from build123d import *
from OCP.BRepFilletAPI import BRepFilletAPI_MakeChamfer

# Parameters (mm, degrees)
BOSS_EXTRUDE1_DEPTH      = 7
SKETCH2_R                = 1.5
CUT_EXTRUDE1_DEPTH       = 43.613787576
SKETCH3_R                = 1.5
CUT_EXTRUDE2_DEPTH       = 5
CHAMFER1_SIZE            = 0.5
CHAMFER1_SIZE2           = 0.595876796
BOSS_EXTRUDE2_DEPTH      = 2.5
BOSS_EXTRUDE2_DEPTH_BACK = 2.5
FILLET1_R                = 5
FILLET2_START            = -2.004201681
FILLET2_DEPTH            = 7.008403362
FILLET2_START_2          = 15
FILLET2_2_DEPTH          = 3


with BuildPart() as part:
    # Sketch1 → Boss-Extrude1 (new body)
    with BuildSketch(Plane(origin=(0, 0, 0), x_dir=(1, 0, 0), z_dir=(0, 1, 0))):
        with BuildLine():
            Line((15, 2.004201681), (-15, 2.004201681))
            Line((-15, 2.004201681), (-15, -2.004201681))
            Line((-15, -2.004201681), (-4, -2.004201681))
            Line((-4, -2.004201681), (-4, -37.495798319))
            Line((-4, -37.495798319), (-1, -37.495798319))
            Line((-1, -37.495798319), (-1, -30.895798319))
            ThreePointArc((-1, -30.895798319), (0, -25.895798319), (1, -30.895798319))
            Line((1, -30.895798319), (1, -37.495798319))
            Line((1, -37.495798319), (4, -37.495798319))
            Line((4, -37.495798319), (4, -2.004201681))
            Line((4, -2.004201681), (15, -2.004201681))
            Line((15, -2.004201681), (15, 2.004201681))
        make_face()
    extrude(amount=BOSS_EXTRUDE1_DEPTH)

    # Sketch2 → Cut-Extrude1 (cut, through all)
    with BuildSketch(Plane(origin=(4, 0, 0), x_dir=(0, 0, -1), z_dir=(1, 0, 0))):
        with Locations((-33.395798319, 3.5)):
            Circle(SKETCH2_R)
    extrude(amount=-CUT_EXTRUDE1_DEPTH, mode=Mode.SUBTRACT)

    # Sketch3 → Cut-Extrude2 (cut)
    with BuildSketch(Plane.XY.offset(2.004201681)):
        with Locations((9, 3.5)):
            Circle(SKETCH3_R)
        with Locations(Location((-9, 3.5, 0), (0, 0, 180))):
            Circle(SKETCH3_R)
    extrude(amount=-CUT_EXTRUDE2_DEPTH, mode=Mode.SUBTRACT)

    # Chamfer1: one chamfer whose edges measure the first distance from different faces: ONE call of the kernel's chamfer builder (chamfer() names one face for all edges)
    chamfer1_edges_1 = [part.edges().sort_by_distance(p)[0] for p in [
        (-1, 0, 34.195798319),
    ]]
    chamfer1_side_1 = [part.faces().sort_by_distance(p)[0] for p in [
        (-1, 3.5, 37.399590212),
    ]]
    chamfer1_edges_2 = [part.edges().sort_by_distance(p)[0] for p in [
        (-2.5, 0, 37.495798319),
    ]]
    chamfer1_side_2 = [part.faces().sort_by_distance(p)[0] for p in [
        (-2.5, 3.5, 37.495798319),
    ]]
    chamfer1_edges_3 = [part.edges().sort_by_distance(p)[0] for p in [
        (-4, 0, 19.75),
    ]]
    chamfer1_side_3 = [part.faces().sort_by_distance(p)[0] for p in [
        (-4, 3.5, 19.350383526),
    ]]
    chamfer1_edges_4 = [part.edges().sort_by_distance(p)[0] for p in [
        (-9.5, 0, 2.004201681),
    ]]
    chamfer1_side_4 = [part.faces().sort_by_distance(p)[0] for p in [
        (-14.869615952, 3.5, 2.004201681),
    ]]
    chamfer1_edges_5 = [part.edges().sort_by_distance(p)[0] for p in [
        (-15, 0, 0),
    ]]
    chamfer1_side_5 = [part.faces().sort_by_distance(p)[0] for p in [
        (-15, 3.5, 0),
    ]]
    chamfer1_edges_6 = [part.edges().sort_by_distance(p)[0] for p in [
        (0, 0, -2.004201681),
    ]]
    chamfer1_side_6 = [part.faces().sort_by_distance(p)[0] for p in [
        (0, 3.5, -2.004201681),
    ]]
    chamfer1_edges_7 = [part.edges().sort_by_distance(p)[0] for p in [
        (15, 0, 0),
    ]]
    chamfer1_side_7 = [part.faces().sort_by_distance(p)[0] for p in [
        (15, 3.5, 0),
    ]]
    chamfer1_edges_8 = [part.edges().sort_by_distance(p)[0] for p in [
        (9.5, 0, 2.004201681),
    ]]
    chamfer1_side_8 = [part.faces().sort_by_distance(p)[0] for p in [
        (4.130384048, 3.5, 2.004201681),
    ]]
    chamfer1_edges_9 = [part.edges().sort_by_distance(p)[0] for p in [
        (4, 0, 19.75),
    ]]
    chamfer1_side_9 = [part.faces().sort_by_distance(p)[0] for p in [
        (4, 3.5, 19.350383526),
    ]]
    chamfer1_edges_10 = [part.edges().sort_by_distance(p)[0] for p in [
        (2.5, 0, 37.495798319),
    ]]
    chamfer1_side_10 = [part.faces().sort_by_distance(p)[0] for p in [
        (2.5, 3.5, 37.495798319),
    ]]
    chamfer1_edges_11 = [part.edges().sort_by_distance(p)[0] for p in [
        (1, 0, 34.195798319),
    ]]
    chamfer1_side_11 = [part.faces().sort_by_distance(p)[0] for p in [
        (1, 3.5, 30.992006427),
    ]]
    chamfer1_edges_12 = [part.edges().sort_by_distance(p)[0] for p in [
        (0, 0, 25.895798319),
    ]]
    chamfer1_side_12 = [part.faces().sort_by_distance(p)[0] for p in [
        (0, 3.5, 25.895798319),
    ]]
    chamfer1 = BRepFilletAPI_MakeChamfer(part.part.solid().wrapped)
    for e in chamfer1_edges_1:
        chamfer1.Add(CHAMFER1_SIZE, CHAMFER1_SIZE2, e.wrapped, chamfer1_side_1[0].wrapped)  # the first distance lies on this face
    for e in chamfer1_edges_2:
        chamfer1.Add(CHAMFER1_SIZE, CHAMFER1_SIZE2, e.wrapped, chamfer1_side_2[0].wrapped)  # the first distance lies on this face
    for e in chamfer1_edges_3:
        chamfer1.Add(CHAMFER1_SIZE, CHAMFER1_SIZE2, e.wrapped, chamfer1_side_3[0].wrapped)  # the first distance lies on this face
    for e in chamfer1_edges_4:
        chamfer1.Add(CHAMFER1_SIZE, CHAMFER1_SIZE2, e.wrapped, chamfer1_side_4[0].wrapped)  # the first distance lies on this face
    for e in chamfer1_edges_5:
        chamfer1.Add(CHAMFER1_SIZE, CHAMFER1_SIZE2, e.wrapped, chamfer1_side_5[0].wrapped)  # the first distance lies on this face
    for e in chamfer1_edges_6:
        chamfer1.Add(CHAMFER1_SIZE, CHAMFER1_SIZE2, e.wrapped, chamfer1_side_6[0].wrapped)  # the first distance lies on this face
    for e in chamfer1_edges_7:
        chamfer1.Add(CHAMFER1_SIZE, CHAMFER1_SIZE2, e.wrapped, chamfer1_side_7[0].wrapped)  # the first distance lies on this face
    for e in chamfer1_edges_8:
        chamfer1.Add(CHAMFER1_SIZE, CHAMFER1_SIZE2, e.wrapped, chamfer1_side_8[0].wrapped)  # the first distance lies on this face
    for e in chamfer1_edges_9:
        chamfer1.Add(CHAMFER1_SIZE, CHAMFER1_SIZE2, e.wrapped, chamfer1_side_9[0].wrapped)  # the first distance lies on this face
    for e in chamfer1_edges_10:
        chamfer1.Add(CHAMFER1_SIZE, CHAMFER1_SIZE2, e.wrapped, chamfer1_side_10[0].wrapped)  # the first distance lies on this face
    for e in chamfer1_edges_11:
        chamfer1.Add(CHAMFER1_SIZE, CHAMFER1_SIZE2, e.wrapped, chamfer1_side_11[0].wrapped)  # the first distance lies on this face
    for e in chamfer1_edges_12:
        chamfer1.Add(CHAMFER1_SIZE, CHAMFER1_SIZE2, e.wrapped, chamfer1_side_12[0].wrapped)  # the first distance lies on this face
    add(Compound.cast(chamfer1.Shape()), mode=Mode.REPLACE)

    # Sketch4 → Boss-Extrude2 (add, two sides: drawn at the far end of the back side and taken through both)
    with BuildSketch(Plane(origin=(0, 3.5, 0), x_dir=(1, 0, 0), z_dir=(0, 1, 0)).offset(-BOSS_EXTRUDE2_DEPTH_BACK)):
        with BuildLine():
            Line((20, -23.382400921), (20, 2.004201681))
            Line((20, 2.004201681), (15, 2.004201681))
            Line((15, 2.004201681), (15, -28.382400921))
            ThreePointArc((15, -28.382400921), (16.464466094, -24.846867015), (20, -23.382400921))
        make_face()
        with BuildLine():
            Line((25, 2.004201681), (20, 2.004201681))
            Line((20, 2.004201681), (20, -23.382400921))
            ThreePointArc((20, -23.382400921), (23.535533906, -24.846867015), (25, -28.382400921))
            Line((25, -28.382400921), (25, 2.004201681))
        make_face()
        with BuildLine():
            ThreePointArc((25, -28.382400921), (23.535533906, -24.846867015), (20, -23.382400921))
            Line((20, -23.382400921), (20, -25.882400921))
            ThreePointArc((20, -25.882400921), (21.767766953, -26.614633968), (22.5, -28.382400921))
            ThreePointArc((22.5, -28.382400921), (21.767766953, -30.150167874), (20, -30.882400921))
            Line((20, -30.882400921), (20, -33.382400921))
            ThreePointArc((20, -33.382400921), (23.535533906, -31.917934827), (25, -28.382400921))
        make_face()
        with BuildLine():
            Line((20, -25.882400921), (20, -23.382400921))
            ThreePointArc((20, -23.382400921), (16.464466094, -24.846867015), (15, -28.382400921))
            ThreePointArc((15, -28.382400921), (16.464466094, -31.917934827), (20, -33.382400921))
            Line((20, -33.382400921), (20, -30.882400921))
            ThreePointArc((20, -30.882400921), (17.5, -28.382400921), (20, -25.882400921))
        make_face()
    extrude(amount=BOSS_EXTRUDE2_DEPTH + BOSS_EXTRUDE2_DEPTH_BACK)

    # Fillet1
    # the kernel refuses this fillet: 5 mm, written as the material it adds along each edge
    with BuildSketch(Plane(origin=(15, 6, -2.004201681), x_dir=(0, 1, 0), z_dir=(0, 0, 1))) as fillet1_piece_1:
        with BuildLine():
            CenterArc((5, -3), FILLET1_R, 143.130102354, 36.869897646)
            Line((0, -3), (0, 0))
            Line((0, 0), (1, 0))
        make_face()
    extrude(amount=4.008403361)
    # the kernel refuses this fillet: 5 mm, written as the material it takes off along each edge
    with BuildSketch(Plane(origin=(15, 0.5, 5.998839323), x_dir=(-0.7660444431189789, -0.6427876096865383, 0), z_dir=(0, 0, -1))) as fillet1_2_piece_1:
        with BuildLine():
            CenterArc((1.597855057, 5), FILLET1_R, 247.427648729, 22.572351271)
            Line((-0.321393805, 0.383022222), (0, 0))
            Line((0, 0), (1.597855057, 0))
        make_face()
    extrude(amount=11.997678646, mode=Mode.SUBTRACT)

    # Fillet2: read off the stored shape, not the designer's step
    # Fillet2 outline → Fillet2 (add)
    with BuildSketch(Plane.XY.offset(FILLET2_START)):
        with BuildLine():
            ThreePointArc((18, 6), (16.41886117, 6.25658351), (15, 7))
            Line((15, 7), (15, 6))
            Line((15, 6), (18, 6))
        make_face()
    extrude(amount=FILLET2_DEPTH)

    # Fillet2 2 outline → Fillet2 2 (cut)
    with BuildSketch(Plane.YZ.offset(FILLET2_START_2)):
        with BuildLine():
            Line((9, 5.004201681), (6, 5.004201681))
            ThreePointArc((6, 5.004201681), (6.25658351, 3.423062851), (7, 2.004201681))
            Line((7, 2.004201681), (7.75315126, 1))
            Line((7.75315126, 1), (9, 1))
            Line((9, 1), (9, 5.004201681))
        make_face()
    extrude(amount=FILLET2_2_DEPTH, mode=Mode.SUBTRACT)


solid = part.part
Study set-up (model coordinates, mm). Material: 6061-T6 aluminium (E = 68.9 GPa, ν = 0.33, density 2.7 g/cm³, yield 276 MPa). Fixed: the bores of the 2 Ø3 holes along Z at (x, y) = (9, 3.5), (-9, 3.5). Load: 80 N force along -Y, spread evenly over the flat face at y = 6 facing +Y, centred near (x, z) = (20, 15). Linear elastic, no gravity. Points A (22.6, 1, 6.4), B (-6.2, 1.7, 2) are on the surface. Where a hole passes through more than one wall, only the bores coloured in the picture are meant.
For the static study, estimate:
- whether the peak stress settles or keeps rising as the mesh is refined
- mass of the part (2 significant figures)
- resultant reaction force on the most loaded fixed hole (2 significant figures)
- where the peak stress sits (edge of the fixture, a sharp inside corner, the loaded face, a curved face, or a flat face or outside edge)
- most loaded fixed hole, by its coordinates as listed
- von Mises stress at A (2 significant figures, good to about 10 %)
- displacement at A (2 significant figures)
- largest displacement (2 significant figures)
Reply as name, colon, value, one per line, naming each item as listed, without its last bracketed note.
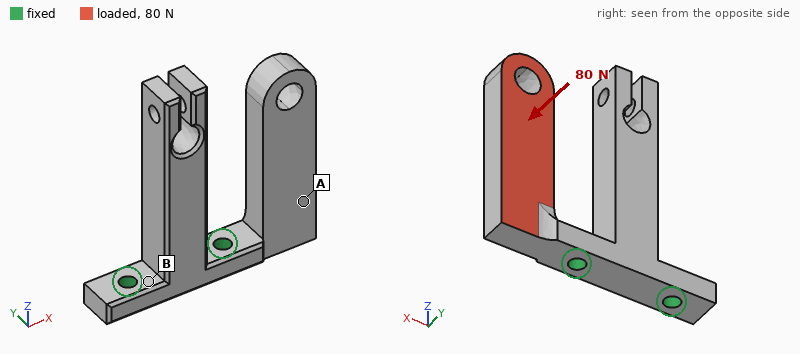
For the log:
whether the peak stress settles or keeps rising as the mesh is refined: keeps rising
mass of the part: 11 g
resultant reaction force on the most loaded fixed hole: 93 N
where the peak stress sits: a sharp inside corner
most loaded fixed hole, by its coordinates as listed: (9, 3.5)
von Mises stress at A: 16 MPa
displacement at A: 0.034 mm
largest displacement: 0.16 mm
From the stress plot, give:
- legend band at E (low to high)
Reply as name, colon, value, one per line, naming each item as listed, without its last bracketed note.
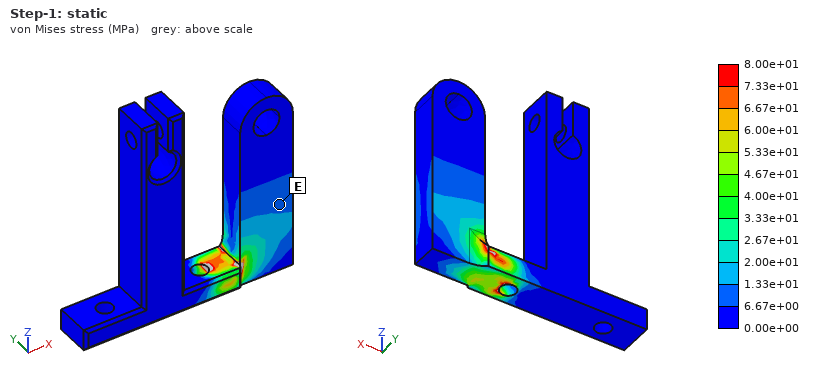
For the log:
legend band at E: 6.67e+00 to 1.33e+01 MPa
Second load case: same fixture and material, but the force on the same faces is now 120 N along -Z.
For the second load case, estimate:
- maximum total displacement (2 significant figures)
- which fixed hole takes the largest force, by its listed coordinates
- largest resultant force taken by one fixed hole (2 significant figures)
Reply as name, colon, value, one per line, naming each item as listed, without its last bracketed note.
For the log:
maximum total displacement: 0.10 mm
which fixed hole takes the largest force, by its listed coordinates: (9, 3.5)
largest resultant force taken by one fixed hole: 120 N
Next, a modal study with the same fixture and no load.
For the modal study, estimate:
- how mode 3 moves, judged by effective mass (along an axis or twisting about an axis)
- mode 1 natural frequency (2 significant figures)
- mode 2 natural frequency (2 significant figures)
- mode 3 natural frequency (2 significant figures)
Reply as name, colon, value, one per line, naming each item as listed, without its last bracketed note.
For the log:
how mode 3 moves, judged by effective mass: along Y
mode 1 natural frequency: 2200 Hz
mode 2 natural frequency: 2200 Hz
mode 3 natural frequency: 3000 Hz
